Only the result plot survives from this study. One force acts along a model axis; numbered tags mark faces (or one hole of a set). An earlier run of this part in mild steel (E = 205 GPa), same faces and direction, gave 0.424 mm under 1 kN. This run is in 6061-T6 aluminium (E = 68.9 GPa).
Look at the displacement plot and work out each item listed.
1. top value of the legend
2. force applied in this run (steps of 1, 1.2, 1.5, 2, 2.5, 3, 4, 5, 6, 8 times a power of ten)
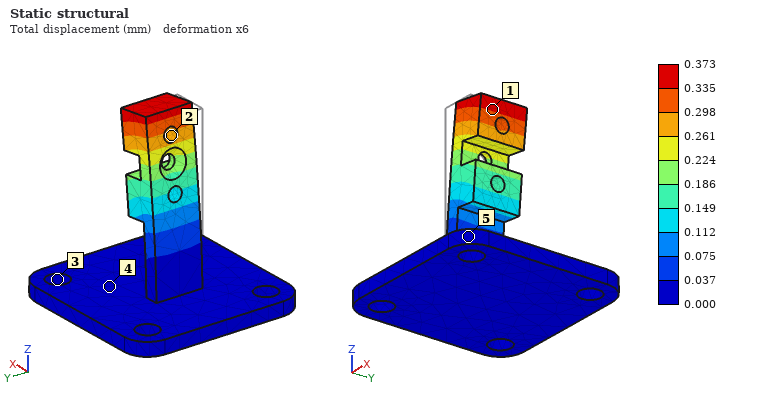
0.373 mm
300 N
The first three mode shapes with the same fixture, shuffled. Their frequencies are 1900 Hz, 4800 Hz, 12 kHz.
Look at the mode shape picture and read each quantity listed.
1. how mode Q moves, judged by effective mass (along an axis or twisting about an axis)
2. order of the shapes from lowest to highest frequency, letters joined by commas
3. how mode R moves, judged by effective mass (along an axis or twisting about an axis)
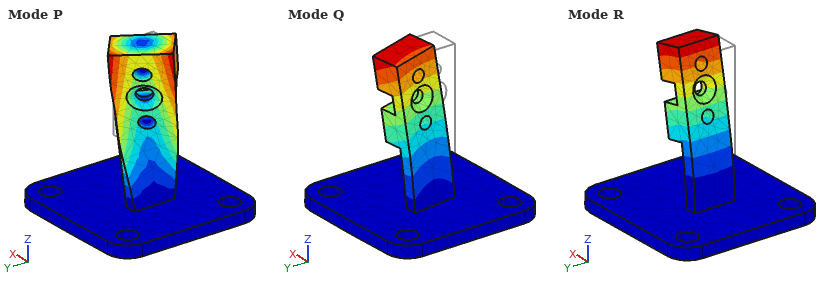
along Y
R, Q, P
along X
